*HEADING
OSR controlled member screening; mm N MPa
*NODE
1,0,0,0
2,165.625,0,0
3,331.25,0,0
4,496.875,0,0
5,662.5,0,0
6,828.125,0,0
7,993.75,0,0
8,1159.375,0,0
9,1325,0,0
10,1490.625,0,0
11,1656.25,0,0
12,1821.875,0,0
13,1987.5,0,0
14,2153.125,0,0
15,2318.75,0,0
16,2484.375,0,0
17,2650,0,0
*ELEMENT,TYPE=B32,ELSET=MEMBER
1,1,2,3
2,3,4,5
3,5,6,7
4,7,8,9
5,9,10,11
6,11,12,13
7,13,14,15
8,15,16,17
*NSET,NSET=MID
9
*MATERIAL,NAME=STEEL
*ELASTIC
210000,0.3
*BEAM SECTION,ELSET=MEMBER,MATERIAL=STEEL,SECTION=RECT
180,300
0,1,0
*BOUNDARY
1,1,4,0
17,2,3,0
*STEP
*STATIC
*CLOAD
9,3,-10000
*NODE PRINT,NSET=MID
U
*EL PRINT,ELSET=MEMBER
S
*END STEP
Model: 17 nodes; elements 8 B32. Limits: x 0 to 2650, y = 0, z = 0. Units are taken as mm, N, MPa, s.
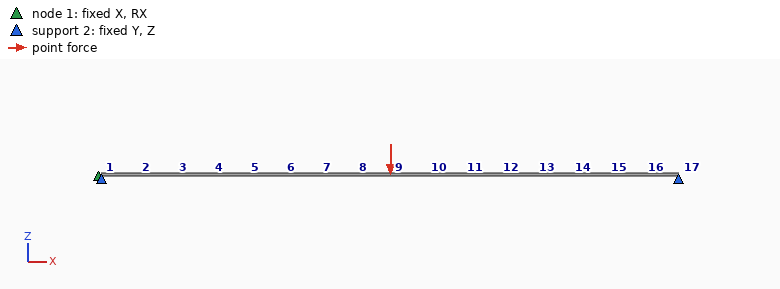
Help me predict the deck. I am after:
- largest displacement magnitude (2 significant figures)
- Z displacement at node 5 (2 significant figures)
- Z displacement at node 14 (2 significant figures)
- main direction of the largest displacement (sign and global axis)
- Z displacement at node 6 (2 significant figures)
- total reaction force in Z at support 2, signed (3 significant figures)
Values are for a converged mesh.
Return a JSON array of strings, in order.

["0.047 mm", "-0.032 mm", "-0.025 mm", "-Z", "-0.038 mm", "10000 N"]
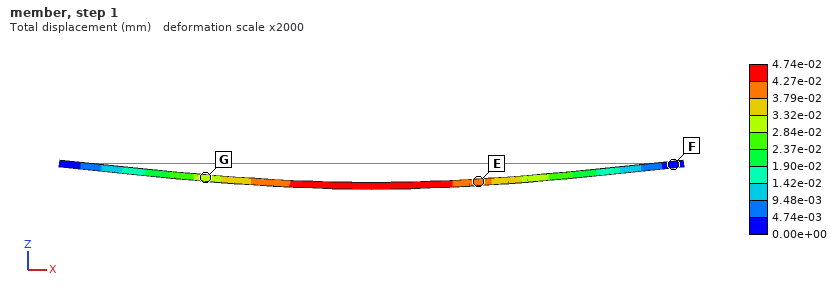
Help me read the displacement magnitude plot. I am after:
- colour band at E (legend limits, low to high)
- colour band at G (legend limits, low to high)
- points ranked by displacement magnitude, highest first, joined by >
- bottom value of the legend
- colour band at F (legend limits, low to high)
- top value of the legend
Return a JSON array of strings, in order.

["3.79e-02 to 4.27e-02 mm", "2.84e-02 to 3.32e-02 mm", "E > G > F", "0.00e+00 mm", "0.00e+00 to 4.74e-03 mm", "4.74e-02 mm"]
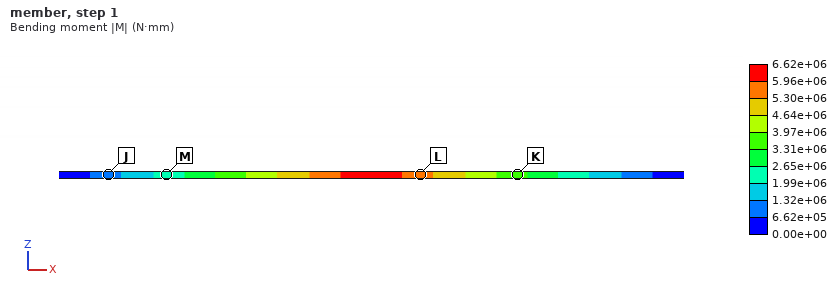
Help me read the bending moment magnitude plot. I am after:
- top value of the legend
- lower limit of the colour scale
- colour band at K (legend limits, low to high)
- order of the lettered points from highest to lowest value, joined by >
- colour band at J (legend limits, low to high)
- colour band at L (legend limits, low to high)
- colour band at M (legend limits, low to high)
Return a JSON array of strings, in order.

["6.62e+06 N·mm", "0.00e+00 N·mm", "3.31e+06 to 3.97e+06 N·mm", "L > K > M > J", "6.62e+05 to 1.32e+06 N·mm", "5.30e+06 to 5.96e+06 N·mm", "1.99e+06 to 2.65e+06 N·mm"]
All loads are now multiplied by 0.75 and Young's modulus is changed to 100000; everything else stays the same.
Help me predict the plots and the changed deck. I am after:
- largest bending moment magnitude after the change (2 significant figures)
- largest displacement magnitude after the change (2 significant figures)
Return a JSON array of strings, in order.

["5.0e+06 N·mm", "0.075 mm"]
